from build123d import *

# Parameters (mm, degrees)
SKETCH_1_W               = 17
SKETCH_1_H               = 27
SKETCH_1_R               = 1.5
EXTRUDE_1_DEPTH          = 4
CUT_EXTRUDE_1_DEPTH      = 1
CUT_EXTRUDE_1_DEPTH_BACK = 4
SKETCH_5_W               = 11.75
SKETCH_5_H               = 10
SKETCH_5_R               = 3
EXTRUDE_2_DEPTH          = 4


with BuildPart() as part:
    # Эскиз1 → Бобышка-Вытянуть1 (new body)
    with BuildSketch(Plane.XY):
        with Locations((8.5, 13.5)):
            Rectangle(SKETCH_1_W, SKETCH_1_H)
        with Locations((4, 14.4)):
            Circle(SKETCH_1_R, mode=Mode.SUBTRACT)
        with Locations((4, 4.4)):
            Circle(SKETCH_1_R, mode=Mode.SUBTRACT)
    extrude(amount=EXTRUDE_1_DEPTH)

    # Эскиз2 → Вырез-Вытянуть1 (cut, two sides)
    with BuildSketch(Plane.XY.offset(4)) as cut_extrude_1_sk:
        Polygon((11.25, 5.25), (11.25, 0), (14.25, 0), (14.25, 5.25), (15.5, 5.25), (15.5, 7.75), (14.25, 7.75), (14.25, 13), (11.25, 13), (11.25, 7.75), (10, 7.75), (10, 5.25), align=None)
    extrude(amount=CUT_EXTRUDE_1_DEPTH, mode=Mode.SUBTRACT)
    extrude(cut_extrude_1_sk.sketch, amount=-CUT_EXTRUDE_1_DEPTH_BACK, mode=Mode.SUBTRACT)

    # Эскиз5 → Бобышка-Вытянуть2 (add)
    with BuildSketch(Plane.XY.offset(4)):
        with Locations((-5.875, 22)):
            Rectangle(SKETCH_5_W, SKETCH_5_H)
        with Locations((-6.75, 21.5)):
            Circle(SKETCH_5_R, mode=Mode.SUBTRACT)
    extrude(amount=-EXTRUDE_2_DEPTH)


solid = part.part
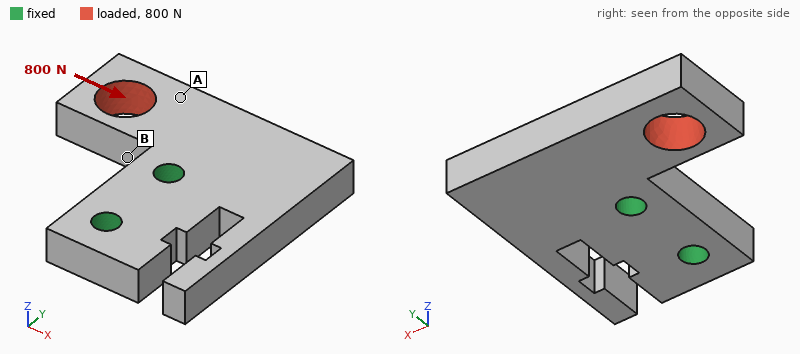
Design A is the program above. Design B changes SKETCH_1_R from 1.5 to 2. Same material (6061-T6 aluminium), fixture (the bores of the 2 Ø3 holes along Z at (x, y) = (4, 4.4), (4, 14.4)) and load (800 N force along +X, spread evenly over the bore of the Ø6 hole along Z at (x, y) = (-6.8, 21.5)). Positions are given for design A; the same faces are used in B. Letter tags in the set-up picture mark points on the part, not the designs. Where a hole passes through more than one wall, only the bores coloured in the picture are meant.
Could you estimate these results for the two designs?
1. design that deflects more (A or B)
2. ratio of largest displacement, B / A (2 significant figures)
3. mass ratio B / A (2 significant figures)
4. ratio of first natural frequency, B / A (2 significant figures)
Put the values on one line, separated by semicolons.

A; 0.84; 0.98; 1.0
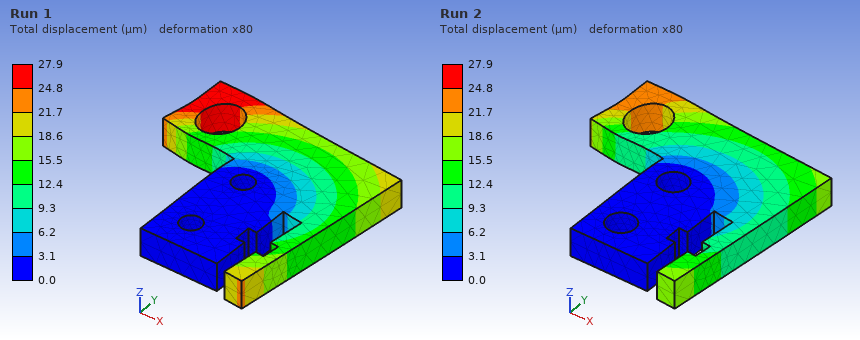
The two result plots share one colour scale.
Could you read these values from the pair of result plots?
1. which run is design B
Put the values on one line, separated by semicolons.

Run 2
